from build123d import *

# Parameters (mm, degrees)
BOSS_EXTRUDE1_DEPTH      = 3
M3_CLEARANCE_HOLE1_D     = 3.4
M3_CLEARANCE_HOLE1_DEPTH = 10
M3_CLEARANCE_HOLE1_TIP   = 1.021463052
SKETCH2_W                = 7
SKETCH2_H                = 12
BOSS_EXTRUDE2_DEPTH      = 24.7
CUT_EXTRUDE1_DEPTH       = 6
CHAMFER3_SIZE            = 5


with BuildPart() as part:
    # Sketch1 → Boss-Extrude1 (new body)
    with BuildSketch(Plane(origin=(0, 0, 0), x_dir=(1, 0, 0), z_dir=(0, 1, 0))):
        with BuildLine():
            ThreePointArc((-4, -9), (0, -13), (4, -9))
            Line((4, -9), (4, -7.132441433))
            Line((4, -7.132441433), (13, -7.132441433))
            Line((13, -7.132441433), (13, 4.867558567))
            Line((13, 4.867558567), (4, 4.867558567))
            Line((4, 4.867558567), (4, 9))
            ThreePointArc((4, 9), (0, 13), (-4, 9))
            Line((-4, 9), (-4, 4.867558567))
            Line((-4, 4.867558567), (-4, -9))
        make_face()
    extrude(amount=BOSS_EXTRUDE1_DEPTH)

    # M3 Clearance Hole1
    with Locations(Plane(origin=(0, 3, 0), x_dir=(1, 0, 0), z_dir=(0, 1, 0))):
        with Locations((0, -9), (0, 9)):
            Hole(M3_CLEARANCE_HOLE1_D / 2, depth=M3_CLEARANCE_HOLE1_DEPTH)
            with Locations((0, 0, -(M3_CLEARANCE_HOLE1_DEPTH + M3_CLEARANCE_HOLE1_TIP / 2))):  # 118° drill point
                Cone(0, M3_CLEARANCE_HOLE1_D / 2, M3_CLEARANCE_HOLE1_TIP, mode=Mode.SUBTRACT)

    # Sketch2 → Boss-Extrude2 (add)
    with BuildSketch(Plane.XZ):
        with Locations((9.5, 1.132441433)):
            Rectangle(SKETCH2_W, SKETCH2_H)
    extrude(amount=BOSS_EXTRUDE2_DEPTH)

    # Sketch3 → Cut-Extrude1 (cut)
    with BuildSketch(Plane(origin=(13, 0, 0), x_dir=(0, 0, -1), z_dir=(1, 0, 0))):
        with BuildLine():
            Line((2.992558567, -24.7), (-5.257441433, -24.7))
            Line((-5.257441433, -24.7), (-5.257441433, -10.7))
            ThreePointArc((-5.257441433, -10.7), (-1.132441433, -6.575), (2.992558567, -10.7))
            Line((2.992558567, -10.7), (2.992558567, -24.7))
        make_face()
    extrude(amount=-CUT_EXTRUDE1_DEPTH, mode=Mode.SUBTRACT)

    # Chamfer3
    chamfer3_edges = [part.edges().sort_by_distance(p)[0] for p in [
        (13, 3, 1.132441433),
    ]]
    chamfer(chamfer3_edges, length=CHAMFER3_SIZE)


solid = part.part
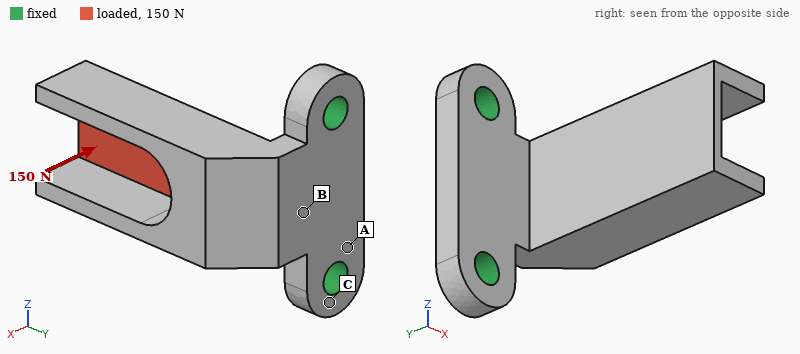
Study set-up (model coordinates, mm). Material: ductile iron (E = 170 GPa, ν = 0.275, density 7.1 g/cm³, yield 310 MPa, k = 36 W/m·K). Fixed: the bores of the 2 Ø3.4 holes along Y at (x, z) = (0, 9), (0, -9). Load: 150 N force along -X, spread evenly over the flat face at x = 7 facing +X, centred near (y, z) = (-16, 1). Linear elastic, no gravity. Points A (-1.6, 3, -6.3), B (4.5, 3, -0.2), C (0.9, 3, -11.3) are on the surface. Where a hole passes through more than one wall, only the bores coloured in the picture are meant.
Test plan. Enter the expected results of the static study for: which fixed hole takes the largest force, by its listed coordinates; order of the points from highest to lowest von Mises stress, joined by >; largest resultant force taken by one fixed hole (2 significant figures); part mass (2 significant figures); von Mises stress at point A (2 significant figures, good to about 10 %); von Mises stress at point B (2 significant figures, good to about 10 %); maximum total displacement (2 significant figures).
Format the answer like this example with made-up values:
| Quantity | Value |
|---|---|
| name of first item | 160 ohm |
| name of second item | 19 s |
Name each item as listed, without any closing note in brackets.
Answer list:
| Quantity | Value |
|---|---|
| which fixed hole takes the largest force, by its listed coordinates | (0, 9) |
| order of the points from highest to lowest von Mises stress, joined by > | B > A > C |
| largest resultant force taken by one fixed hole | 90 N |
| part mass | 14 g |
| von Mises stress at point A | 49 MPa |
| von Mises stress at point B | 110 MPa |
| maximum total displacement | 0.14 mm |
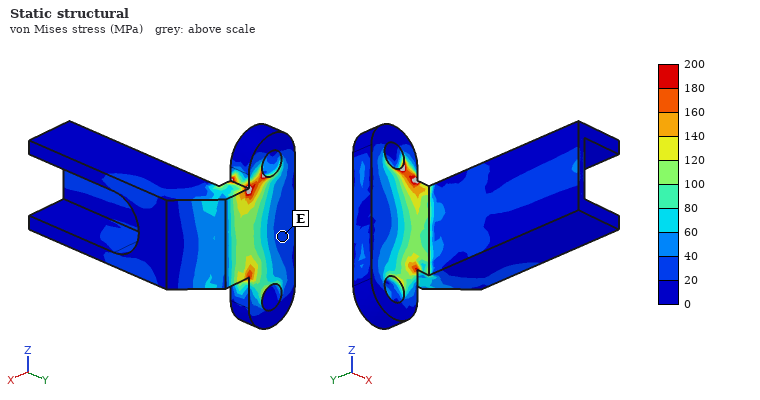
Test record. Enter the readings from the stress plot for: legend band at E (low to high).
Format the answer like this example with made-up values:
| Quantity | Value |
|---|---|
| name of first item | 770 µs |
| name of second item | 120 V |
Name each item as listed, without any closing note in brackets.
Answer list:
| Quantity | Value |
|---|---|
| legend band at E | 20 to 40 MPa |
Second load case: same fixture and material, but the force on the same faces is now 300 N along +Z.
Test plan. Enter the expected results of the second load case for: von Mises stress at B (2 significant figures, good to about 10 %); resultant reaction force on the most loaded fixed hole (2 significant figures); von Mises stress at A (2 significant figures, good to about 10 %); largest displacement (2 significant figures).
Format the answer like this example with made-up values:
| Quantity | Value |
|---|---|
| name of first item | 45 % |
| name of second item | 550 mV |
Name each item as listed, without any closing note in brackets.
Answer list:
| Quantity | Value |
|---|---|
| von Mises stress at B | 100 MPa |
| resultant reaction force on the most loaded fixed hole | 440 N |
| von Mises stress at A | 44 MPa |
| largest displacement | 84 µm |
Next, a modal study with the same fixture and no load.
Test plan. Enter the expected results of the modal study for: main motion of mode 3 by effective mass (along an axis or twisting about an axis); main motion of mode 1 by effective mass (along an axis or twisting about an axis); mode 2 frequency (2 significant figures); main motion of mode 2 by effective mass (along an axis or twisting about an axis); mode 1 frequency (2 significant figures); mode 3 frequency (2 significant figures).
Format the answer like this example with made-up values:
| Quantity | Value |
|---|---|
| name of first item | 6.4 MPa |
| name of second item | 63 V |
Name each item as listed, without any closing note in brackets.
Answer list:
| Quantity | Value |
|---|---|
| main motion of mode 3 by effective mass | along Y |
| main motion of mode 1 by effective mass | along X |
| mode 2 frequency | 5100 Hz |
| main motion of mode 2 by effective mass | along Z |
| mode 1 frequency | 2700 Hz |
| mode 3 frequency | 12 kHz |
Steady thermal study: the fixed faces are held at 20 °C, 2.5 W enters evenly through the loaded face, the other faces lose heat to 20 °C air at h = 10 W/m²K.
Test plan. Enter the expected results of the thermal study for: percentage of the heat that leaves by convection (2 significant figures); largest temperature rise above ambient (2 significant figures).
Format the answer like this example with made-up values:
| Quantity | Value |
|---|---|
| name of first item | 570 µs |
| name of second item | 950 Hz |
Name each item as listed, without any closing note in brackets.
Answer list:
| Quantity | Value |
|---|---|
| percentage of the heat that leaves by convection | 13 % |
| largest temperature rise above ambient | 41 K |
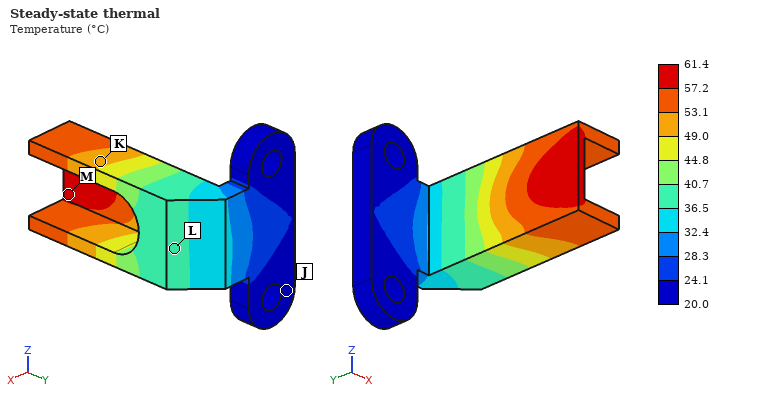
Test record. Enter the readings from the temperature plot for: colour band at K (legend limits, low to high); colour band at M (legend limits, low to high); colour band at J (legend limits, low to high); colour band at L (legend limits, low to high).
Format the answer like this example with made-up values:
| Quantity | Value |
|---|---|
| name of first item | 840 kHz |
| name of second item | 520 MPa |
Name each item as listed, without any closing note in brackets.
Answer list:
| Quantity | Value |
|---|---|
| colour band at K | 49.0 to 53.1 °C |
| colour band at M | 57.2 to 61.4 °C |
| colour band at J | 20.0 to 24.1 °C |
| colour band at L | 36.5 to 40.7 °C |
